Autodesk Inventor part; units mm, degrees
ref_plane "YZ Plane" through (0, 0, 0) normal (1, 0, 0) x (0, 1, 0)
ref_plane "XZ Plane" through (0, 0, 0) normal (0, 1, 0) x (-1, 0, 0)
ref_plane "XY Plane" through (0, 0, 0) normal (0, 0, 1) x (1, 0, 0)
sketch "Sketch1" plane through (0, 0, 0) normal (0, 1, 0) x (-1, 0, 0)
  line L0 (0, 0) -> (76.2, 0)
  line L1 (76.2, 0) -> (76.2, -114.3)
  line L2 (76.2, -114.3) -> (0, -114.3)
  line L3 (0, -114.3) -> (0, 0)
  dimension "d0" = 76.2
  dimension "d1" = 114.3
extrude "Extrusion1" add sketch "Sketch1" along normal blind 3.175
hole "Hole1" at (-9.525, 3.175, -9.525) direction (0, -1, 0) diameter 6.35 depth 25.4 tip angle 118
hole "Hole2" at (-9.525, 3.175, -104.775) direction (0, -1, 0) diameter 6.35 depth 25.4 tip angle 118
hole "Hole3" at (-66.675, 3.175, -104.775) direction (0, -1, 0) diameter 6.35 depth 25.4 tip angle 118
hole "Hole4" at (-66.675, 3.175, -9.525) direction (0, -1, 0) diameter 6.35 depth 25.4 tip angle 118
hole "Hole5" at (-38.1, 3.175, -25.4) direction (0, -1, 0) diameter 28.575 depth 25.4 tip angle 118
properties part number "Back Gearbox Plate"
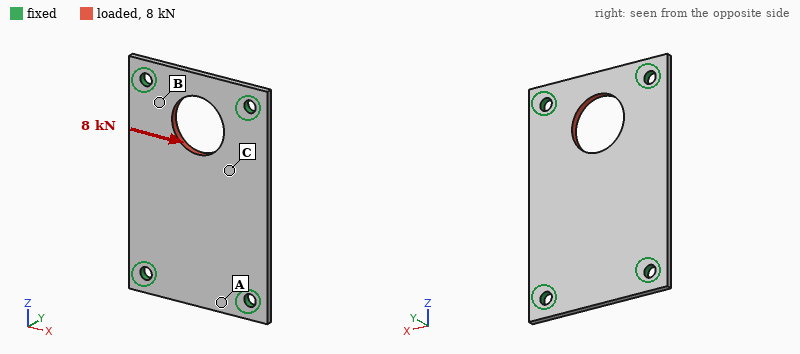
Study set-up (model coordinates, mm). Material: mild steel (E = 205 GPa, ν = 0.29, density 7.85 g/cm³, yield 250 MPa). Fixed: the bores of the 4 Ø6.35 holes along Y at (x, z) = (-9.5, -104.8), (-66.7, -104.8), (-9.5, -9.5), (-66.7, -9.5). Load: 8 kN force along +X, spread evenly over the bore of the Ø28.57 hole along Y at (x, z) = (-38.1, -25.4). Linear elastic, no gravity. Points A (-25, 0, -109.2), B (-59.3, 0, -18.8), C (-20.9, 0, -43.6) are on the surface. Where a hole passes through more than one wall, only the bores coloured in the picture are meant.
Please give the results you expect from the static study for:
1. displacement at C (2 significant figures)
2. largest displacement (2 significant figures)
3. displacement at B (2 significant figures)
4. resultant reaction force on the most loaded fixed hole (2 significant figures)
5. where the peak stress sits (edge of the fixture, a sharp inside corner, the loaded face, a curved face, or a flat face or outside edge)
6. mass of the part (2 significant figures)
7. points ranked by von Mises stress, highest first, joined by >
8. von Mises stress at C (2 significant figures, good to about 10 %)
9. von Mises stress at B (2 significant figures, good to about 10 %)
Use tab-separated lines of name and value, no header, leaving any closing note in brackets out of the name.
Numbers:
displacement at C	11 µm
largest displacement	12 µm
displacement at B	5.0 µm
resultant reaction force on the most loaded fixed hole	3.1 kN
where the peak stress sits	edge of the fixture
mass of the part	200 g
points ranked by von Mises stress, highest first, joined by >	B > C > A
von Mises stress at C	19 MPa
von Mises stress at B	47 MPa
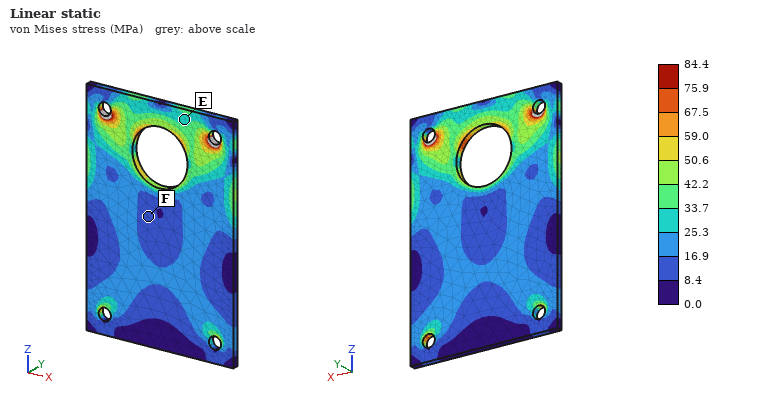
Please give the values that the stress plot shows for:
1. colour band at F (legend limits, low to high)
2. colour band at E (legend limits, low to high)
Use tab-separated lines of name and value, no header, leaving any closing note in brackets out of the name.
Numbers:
colour band at F	8.4 to 16.9 MPa
colour band at E	25.3 to 33.7 MPa
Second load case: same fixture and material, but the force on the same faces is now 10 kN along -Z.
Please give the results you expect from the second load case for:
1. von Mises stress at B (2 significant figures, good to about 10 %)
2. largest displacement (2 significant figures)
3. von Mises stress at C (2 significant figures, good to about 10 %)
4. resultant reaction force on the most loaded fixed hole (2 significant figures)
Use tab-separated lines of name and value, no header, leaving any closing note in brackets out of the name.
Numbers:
von Mises stress at B	59 MPa
largest displacement	18 µm
von Mises stress at C	34 MPa
resultant reaction force on the most loaded fixed hole	3.5 kN
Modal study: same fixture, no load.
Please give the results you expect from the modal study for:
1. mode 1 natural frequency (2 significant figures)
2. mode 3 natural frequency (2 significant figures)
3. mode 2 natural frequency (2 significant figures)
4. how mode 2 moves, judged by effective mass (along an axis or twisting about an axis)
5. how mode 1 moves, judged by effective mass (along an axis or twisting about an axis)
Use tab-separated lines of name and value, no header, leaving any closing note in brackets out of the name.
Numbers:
mode 1 natural frequency	1700 Hz
mode 3 natural frequency	4200 Hz
mode 2 natural frequency	2400 Hz
how mode 2 moves, judged by effective mass	twisting about Z
how mode 1 moves, judged by effective mass	along Y
